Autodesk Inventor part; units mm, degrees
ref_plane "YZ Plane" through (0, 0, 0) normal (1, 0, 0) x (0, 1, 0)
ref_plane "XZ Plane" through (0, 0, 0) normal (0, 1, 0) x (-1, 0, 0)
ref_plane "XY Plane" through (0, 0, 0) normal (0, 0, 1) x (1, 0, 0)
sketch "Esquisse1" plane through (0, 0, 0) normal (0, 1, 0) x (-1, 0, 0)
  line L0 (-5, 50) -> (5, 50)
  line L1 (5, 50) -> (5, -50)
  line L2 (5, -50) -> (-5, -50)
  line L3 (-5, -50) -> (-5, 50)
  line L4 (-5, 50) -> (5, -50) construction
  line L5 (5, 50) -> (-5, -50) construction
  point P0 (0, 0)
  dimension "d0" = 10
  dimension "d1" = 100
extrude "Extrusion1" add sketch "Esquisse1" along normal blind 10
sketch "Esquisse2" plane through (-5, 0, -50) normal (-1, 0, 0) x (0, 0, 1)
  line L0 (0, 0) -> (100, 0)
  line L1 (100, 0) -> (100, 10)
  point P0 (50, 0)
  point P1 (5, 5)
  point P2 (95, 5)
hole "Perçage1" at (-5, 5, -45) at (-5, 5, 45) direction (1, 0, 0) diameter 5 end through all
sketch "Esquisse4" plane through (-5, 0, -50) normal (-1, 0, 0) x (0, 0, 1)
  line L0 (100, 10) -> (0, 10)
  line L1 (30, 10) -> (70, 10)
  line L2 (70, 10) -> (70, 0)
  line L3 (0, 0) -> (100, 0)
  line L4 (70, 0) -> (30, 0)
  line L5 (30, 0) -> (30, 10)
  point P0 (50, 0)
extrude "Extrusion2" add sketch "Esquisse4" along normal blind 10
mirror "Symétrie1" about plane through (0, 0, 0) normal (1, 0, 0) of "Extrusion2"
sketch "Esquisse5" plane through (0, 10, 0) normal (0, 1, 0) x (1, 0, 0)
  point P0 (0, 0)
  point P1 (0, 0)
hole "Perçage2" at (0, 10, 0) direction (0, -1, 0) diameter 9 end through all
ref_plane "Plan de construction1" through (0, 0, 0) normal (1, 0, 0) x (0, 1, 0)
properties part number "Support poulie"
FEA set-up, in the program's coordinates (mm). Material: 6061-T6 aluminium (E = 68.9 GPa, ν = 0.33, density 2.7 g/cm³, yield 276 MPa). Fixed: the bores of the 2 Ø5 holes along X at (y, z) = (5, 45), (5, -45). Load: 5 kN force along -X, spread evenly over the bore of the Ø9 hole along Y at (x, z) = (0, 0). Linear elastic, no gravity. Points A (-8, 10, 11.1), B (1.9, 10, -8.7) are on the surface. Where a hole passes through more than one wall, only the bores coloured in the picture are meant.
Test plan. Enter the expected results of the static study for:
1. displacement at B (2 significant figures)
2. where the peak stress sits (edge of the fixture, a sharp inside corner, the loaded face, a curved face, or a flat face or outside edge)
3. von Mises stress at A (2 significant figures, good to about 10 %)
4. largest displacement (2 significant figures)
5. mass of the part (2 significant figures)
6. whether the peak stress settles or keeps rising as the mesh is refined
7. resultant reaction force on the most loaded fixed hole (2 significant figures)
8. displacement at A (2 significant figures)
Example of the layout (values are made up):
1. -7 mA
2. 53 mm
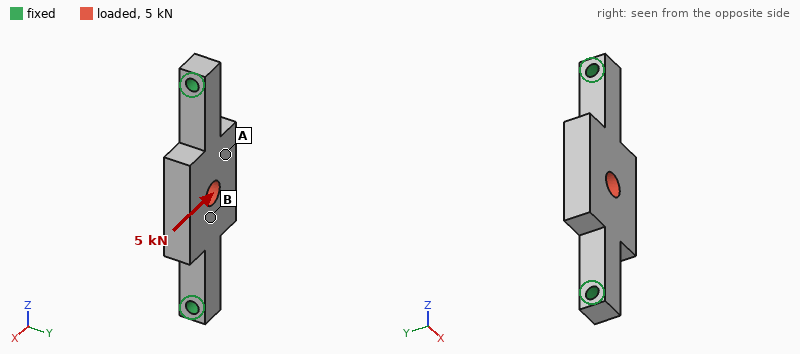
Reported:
1. 0.11 mm
2. edge of the fixture
3. 39 MPa
4. 0.11 mm
5. 46 g
6. keeps rising
7. 2.5 kN
8. 0.11 mm
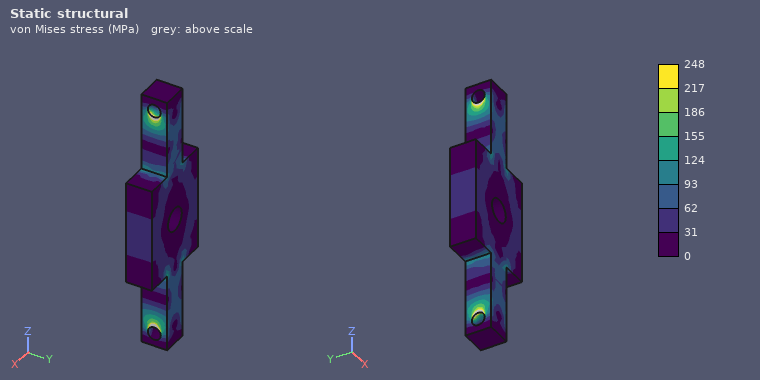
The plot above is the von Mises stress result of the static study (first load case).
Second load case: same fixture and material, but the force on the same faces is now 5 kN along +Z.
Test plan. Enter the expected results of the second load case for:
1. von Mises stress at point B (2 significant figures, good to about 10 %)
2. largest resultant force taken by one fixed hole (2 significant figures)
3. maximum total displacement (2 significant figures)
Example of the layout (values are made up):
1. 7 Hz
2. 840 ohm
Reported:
1. 20 MPa
2. 2.5 kN
3. 13 µm
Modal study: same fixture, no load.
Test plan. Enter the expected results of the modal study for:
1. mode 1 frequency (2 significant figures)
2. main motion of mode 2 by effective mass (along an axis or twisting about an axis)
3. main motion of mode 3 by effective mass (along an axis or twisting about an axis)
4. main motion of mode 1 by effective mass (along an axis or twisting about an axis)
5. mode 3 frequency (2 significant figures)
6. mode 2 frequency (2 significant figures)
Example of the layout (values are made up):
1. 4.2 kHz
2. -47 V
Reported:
1. 4200 Hz
2. twisting about Z
3. along X
4. along Y
5. 6000 Hz
6. 5100 Hz
